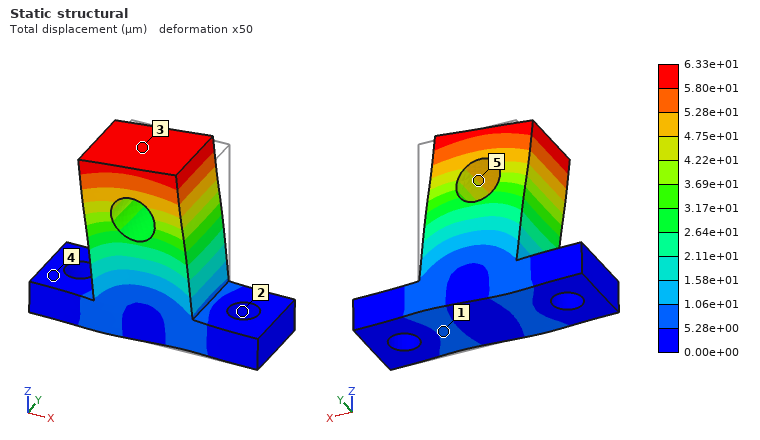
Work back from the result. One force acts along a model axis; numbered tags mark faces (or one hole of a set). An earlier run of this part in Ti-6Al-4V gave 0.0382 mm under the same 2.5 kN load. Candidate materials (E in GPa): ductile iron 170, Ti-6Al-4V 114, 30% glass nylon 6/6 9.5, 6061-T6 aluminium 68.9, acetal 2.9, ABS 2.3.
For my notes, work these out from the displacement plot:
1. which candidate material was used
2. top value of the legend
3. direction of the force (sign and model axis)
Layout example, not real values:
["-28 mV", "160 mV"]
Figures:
["6061-T6 aluminium", "6.33e+01 µm", "-X"]
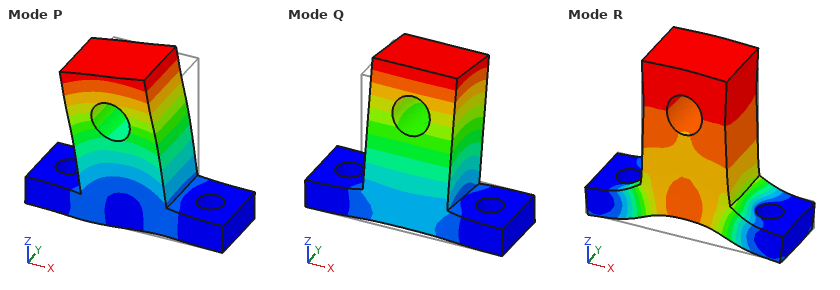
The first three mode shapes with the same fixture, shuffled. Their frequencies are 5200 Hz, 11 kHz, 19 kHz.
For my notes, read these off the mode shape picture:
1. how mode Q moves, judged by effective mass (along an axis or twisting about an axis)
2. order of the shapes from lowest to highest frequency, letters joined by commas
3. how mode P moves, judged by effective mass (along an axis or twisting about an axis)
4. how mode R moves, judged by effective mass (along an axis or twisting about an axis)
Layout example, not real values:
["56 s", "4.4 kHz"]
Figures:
["along Y", "Q, P, R", "along X", "along Z"]
